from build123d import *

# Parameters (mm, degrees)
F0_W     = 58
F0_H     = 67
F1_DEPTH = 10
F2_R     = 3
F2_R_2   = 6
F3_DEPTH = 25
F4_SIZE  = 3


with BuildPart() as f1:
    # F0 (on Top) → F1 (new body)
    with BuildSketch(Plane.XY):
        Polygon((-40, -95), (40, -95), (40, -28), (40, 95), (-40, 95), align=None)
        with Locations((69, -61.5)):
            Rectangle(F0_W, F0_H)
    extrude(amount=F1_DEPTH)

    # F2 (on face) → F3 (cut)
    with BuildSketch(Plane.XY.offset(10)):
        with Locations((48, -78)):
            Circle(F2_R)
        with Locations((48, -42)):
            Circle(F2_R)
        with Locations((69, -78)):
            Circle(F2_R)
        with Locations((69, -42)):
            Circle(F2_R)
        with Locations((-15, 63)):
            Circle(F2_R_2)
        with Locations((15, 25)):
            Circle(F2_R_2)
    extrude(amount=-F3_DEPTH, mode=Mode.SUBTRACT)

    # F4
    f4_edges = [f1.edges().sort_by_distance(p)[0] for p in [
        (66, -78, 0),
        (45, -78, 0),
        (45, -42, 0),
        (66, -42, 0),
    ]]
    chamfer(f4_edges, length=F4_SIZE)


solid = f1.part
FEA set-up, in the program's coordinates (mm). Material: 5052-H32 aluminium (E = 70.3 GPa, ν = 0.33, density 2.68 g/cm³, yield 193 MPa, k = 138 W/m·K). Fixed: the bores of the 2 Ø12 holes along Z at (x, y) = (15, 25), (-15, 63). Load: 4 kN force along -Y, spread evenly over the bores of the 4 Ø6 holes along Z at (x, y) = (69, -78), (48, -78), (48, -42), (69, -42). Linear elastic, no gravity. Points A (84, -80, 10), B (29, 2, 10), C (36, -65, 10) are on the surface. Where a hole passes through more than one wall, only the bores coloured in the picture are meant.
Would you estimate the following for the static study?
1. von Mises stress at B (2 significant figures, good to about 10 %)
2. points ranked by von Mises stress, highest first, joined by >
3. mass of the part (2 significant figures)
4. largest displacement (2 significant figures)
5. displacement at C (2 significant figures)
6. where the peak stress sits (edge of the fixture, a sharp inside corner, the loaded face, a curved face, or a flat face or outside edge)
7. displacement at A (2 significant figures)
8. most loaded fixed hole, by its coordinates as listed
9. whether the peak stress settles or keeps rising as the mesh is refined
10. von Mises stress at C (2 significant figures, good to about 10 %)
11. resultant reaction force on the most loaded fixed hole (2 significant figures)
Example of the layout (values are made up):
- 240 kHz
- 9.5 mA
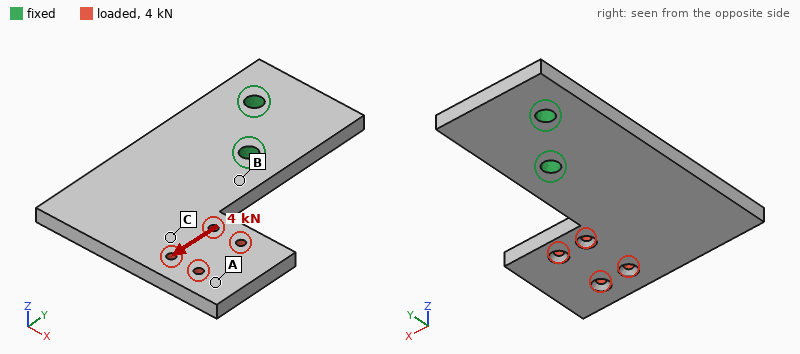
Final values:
- 25 MPa
- B > C > A
- 500 g
- 0.16 mm
- 0.084 mm
- edge of the fixture
- 0.14 mm
- (15, 25)
- keeps rising
- 12 MPa
- 6.6 kN
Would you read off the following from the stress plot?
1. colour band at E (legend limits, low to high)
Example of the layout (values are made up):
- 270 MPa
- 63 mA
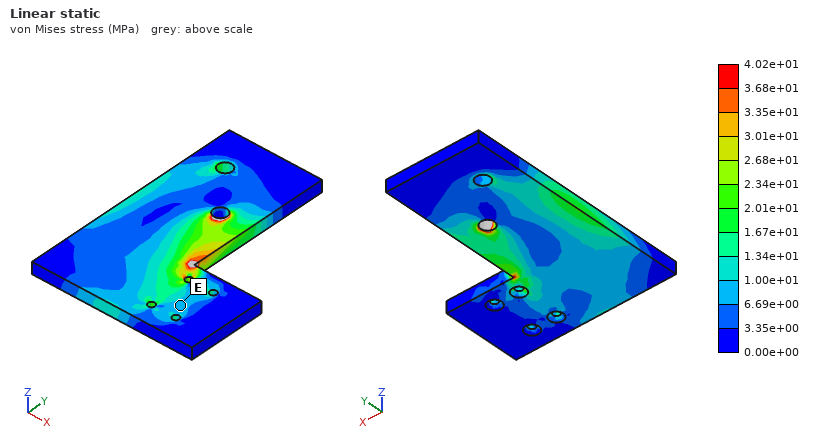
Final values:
- 6.69e+00 to 1.00e+01 MPa
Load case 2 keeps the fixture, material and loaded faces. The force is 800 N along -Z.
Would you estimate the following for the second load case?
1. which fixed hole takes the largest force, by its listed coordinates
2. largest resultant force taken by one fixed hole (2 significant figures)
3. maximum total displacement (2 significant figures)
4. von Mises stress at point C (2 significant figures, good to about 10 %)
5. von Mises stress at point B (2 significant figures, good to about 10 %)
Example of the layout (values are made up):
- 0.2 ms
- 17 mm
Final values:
- (15, 25)
- 1.5 kN
- 1.0 mm
- 14 MPa
- 49 MPa
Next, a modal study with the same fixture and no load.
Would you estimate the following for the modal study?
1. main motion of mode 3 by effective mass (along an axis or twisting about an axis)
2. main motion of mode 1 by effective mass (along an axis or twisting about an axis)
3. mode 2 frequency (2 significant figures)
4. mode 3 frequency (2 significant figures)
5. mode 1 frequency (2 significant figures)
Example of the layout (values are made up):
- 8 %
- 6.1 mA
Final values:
- along X
- along Z
- 730 Hz
- 1900 Hz
- 420 Hz
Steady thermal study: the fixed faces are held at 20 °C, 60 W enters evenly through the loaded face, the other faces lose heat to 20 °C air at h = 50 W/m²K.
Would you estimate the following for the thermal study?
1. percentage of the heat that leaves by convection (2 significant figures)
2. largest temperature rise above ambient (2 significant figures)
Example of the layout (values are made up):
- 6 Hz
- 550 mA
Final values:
- 57 %
- 41 K
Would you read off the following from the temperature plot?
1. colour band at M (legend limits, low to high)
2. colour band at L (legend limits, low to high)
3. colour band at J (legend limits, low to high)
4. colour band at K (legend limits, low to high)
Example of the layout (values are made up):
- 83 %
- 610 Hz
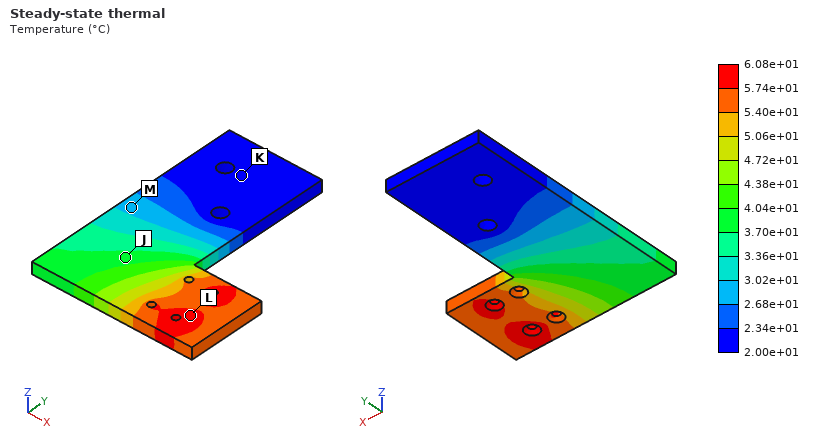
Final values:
- 2.68e+01 to 3.02e+01 °C
- 5.74e+01 to 6.08e+01 °C
- 3.70e+01 to 4.04e+01 °C
- 2.00e+01 to 2.34e+01 °C
